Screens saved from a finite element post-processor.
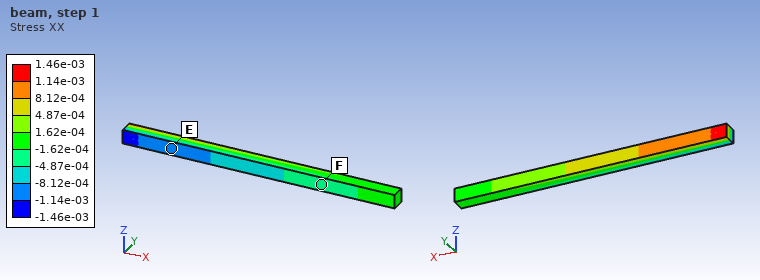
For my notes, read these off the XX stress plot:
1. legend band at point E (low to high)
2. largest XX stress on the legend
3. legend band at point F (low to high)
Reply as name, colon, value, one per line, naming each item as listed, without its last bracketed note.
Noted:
legend band at point E: -1.14e-03 to -8.12e-04
largest XX stress on the legend: 1.46e-03
legend band at point F: -4.87e-04 to -1.62e-04
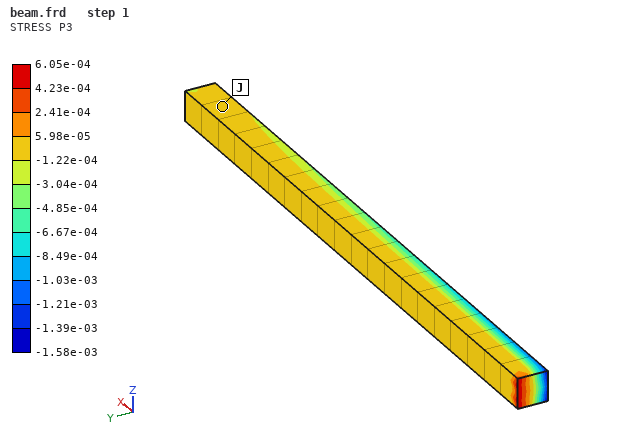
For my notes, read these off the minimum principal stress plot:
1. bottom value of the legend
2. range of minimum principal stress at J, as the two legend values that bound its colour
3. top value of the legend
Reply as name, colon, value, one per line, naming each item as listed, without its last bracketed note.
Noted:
bottom value of the legend: -1.58e-03
range of minimum principal stress at J, as the two legend values that bound its colour: -1.22e-04 to 5.98e-05
top value of the legend: 6.05e-04
